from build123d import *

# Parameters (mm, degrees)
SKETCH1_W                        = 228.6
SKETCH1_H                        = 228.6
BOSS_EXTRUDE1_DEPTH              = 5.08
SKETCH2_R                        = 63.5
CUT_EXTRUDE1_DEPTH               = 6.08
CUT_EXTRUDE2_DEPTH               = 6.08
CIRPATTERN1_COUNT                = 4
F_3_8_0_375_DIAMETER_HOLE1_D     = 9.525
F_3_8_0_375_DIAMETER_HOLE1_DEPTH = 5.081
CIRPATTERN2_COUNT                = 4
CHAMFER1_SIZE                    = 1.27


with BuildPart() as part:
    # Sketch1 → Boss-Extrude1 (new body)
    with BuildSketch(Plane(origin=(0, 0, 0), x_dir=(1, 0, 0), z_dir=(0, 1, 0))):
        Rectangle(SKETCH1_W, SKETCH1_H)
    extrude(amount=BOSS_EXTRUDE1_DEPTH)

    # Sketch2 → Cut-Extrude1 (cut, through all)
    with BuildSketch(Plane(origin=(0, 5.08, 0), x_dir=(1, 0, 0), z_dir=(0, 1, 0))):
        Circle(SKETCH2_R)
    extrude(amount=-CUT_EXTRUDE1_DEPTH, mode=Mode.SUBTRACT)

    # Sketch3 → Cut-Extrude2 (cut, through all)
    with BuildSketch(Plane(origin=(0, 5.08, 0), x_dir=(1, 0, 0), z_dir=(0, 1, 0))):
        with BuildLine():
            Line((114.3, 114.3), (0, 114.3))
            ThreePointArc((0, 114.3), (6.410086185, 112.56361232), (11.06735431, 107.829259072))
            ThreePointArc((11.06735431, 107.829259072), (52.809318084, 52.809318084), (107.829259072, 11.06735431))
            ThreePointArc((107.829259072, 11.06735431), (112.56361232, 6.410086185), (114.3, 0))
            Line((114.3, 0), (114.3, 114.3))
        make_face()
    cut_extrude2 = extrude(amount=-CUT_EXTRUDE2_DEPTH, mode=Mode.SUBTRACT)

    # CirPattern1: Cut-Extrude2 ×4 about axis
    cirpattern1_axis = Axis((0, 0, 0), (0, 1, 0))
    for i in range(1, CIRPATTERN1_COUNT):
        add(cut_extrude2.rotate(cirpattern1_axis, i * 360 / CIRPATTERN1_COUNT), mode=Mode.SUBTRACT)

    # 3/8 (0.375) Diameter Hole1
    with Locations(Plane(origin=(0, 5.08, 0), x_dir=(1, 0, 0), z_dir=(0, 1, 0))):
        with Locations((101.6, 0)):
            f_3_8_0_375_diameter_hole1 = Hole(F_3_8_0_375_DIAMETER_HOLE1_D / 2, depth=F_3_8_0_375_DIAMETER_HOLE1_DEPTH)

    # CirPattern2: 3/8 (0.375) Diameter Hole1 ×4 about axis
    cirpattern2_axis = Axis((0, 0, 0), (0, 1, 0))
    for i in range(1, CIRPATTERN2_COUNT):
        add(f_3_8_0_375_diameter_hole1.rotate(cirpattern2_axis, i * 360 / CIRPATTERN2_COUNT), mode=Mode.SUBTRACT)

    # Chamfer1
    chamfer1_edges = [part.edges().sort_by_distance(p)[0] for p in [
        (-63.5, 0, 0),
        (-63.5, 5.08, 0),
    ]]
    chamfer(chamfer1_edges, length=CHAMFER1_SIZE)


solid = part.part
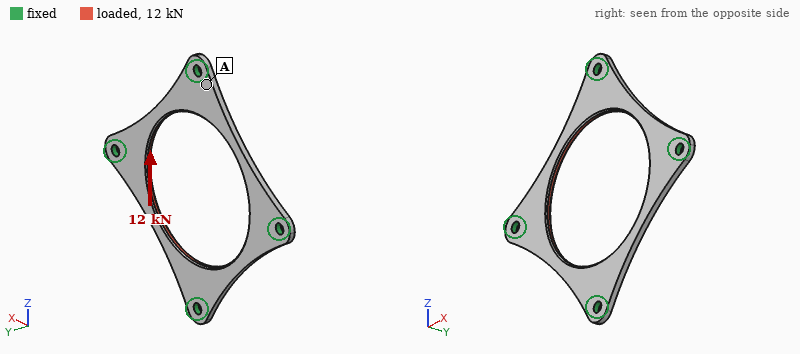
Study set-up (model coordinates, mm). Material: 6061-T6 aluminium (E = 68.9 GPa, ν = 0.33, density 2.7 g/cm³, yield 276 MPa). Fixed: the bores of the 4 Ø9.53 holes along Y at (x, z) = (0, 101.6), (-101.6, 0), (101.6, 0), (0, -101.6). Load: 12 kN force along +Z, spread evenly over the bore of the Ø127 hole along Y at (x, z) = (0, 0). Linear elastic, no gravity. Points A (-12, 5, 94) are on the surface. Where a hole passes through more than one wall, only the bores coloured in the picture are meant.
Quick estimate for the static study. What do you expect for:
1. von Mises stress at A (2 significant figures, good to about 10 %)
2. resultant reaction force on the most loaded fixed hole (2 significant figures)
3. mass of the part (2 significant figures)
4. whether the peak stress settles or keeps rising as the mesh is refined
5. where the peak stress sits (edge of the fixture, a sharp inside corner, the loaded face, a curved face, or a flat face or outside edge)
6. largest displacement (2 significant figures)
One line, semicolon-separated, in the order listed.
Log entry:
27 MPa; 3.6 kN; 160 g; keeps rising; edge of the fixture; 0.10 mm
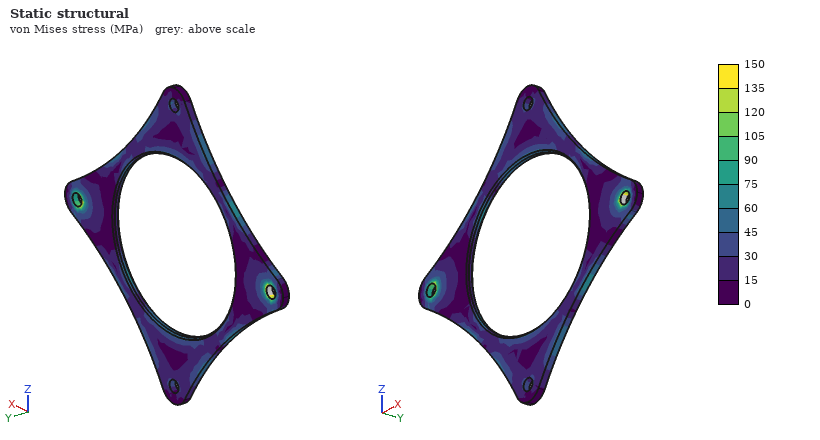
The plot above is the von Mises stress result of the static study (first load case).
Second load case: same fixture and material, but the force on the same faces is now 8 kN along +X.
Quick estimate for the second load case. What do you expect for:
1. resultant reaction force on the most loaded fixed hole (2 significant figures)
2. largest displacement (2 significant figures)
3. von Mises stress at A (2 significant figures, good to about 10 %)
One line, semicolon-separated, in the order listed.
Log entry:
2.4 kN; 70 µm; 20 MPa
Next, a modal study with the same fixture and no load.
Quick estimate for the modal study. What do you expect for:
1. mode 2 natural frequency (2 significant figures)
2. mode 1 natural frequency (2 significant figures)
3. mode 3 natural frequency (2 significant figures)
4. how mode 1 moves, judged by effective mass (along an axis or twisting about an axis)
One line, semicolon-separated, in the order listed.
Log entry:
1700 Hz; 1700 Hz; 1700 Hz; along Y
